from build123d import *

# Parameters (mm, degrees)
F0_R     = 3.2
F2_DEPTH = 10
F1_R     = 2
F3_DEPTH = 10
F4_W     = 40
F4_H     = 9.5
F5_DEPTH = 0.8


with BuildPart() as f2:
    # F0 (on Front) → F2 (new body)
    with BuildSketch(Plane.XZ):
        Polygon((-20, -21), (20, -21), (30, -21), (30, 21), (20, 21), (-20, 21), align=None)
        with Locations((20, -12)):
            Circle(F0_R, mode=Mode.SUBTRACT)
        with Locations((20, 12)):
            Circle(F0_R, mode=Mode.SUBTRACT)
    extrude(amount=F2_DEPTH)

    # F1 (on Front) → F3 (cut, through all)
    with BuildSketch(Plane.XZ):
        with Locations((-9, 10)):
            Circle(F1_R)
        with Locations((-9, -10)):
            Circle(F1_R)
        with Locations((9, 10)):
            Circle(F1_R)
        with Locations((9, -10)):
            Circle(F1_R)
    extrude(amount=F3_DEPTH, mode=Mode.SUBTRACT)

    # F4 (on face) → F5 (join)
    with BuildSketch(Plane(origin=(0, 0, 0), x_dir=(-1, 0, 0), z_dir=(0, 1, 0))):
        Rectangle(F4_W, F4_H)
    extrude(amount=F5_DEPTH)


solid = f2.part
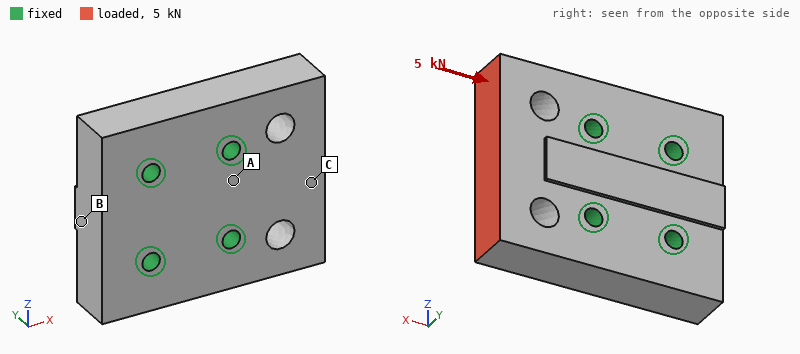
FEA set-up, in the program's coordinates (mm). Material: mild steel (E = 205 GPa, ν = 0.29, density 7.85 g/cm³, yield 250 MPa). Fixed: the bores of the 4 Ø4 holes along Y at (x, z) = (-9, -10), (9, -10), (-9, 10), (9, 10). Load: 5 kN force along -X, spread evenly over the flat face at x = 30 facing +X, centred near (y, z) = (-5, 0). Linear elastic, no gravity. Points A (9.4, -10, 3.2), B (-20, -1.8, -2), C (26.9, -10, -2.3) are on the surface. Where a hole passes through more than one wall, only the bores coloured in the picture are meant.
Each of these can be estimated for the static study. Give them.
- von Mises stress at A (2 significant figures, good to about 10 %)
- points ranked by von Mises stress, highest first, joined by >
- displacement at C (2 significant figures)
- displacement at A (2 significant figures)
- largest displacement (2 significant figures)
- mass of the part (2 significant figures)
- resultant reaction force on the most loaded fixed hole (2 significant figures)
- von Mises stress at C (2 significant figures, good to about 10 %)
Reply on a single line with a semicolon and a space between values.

7.8 MPa; C > A > B; 1.3 µm; 0.40 µm; 2.1 µm; 160 g; 2.0 kN; 14 MPa
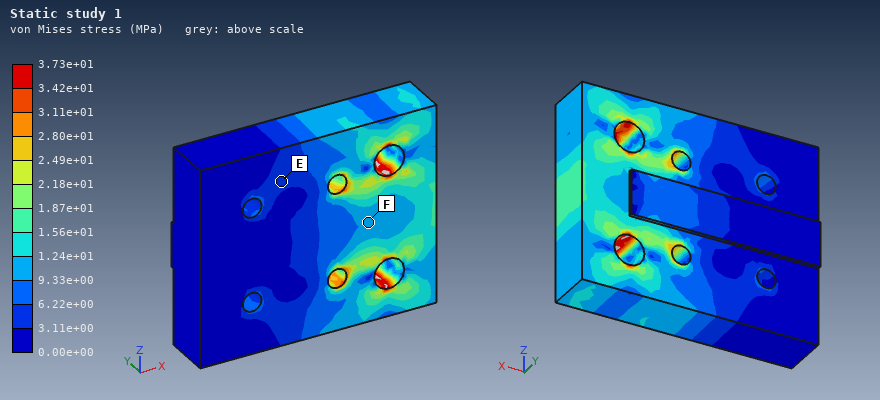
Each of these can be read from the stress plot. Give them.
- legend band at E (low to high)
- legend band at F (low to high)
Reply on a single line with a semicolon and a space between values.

3.11e+00 to 6.22e+00 MPa; 9.33e+00 to 1.24e+01 MPa
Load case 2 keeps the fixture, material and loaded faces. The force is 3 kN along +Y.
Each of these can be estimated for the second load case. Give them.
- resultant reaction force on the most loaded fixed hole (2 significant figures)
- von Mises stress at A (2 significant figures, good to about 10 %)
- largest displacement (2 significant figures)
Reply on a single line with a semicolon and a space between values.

2.0 kN; 49 MPa; 20 µm
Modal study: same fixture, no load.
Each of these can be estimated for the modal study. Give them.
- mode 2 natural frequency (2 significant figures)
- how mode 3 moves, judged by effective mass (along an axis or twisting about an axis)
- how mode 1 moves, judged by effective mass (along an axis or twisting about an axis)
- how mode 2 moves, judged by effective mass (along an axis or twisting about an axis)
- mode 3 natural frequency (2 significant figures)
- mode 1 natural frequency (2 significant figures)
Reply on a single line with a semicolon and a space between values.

20 kHz; along Z; along Y; twisting about X; 26 kHz; 15 kHz
